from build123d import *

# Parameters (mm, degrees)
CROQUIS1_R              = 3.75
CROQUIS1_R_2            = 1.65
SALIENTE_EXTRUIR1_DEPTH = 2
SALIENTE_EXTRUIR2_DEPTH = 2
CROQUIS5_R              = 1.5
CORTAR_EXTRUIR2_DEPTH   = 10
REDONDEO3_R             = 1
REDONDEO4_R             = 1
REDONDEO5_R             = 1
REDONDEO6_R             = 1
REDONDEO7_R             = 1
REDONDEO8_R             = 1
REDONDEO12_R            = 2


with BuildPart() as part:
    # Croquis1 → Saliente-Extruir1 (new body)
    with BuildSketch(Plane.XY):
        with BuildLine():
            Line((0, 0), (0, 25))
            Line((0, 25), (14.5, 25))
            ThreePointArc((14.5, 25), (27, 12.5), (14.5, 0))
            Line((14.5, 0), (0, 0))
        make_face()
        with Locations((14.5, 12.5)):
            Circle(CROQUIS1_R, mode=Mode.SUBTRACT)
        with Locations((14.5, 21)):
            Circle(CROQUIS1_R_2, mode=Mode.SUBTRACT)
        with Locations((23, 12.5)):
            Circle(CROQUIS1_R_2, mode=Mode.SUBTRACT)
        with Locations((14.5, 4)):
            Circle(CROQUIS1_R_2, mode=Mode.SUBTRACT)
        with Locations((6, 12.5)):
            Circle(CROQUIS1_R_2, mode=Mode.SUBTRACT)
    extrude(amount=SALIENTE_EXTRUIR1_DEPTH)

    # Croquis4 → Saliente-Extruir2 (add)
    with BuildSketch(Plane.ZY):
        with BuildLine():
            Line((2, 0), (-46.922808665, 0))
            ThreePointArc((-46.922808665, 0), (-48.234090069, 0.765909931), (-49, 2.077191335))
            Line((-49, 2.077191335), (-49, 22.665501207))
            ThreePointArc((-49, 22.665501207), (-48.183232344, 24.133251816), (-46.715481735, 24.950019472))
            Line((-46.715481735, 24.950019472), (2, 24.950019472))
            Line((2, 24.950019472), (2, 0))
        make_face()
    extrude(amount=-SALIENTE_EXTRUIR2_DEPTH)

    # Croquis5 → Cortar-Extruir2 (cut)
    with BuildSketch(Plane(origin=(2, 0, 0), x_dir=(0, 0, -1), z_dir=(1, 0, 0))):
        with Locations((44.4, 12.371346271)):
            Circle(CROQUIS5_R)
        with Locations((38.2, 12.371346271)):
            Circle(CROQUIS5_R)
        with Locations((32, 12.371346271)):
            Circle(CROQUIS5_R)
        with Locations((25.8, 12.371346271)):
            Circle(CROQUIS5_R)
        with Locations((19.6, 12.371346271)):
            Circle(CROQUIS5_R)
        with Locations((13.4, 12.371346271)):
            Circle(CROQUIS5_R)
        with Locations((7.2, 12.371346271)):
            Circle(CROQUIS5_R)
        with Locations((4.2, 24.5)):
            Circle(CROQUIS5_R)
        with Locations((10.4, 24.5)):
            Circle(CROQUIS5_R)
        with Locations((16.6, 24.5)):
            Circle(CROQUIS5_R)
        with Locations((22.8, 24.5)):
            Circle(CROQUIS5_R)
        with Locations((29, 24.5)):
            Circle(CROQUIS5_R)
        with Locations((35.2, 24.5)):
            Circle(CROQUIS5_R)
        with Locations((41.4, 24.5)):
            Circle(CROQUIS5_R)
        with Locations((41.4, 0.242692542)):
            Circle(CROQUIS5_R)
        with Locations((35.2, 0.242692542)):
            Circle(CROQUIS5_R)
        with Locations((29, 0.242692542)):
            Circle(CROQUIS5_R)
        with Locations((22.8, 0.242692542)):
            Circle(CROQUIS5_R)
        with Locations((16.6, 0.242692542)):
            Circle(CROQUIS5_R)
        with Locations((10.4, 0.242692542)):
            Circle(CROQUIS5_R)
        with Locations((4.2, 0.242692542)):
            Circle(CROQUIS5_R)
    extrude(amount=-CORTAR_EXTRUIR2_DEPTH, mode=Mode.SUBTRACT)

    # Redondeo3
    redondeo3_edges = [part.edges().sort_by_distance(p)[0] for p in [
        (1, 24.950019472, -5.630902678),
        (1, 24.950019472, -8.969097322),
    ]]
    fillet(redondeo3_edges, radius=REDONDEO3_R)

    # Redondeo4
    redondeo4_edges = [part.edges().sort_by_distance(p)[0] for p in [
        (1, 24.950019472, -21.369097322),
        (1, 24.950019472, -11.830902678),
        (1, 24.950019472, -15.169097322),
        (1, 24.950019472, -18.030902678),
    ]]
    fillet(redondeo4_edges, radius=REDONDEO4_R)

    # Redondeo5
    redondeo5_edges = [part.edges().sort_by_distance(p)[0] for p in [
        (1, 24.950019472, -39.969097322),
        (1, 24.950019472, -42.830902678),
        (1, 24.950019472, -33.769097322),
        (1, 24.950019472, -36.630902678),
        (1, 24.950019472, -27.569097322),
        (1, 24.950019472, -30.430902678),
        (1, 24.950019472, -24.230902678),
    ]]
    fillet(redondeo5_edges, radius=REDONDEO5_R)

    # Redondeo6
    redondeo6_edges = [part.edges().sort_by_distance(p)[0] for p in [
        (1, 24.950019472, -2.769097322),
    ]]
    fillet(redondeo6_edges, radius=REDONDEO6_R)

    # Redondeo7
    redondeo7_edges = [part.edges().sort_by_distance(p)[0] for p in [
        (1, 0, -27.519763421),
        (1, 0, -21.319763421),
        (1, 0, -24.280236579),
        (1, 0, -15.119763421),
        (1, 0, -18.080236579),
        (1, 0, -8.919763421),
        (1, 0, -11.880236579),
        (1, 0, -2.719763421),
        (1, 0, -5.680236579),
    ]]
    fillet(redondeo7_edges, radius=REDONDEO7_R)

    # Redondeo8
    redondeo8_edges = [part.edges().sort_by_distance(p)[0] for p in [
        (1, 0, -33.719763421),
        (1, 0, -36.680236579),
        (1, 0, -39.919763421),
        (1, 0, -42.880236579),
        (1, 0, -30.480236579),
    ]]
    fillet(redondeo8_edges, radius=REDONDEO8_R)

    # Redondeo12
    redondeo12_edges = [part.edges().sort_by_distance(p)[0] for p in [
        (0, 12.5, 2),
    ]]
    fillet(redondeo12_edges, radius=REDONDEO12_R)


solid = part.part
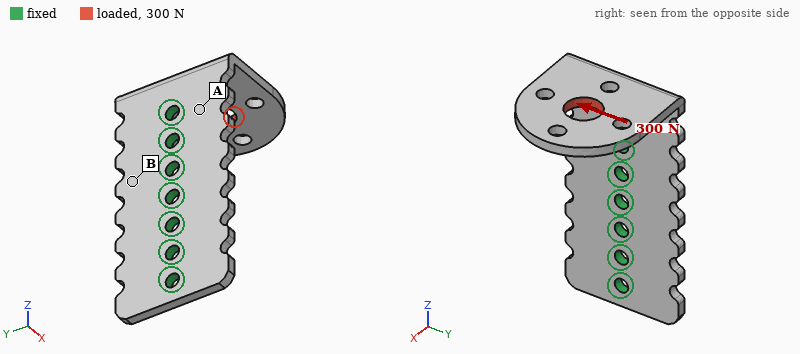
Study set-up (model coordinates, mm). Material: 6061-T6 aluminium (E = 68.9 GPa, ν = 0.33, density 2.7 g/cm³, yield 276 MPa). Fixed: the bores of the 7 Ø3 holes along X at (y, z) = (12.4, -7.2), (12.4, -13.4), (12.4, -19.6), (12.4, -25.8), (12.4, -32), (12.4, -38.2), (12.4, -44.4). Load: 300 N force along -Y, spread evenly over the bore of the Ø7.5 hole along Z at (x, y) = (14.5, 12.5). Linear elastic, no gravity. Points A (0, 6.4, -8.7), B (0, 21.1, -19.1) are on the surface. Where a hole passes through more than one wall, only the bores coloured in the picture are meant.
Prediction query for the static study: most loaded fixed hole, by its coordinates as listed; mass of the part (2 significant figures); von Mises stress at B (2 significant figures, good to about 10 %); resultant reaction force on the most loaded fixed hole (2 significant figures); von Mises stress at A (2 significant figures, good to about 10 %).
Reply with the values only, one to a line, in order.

(12.4, -7.2)
8.8 g
36 MPa
390 N
130 MPa
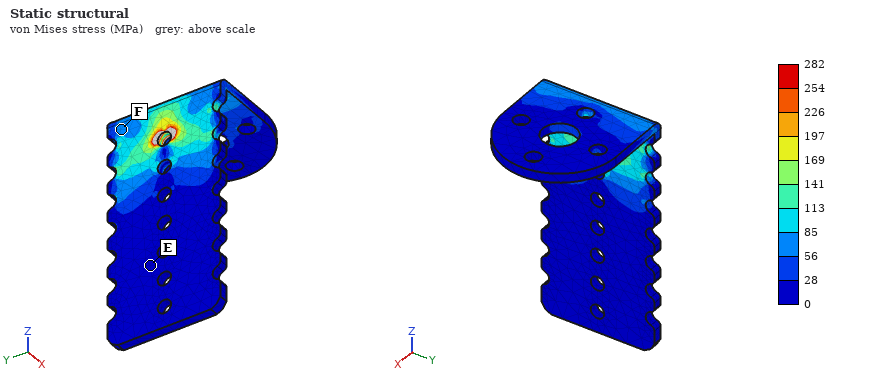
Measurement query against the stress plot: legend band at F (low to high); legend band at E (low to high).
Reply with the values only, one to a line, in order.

56 to 85 MPa
0 to 28 MPa
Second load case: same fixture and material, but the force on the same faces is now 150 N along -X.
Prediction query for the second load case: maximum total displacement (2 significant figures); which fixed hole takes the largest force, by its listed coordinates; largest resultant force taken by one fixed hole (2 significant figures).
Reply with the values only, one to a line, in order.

0.13 mm
(12.4, -7.2)
210 N
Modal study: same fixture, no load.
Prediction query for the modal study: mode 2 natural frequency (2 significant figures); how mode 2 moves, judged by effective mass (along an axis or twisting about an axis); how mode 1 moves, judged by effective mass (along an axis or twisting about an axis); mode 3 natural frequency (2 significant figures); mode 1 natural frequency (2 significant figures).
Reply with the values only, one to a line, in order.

2900 Hz
along Y
along Z
6600 Hz
1900 Hz
